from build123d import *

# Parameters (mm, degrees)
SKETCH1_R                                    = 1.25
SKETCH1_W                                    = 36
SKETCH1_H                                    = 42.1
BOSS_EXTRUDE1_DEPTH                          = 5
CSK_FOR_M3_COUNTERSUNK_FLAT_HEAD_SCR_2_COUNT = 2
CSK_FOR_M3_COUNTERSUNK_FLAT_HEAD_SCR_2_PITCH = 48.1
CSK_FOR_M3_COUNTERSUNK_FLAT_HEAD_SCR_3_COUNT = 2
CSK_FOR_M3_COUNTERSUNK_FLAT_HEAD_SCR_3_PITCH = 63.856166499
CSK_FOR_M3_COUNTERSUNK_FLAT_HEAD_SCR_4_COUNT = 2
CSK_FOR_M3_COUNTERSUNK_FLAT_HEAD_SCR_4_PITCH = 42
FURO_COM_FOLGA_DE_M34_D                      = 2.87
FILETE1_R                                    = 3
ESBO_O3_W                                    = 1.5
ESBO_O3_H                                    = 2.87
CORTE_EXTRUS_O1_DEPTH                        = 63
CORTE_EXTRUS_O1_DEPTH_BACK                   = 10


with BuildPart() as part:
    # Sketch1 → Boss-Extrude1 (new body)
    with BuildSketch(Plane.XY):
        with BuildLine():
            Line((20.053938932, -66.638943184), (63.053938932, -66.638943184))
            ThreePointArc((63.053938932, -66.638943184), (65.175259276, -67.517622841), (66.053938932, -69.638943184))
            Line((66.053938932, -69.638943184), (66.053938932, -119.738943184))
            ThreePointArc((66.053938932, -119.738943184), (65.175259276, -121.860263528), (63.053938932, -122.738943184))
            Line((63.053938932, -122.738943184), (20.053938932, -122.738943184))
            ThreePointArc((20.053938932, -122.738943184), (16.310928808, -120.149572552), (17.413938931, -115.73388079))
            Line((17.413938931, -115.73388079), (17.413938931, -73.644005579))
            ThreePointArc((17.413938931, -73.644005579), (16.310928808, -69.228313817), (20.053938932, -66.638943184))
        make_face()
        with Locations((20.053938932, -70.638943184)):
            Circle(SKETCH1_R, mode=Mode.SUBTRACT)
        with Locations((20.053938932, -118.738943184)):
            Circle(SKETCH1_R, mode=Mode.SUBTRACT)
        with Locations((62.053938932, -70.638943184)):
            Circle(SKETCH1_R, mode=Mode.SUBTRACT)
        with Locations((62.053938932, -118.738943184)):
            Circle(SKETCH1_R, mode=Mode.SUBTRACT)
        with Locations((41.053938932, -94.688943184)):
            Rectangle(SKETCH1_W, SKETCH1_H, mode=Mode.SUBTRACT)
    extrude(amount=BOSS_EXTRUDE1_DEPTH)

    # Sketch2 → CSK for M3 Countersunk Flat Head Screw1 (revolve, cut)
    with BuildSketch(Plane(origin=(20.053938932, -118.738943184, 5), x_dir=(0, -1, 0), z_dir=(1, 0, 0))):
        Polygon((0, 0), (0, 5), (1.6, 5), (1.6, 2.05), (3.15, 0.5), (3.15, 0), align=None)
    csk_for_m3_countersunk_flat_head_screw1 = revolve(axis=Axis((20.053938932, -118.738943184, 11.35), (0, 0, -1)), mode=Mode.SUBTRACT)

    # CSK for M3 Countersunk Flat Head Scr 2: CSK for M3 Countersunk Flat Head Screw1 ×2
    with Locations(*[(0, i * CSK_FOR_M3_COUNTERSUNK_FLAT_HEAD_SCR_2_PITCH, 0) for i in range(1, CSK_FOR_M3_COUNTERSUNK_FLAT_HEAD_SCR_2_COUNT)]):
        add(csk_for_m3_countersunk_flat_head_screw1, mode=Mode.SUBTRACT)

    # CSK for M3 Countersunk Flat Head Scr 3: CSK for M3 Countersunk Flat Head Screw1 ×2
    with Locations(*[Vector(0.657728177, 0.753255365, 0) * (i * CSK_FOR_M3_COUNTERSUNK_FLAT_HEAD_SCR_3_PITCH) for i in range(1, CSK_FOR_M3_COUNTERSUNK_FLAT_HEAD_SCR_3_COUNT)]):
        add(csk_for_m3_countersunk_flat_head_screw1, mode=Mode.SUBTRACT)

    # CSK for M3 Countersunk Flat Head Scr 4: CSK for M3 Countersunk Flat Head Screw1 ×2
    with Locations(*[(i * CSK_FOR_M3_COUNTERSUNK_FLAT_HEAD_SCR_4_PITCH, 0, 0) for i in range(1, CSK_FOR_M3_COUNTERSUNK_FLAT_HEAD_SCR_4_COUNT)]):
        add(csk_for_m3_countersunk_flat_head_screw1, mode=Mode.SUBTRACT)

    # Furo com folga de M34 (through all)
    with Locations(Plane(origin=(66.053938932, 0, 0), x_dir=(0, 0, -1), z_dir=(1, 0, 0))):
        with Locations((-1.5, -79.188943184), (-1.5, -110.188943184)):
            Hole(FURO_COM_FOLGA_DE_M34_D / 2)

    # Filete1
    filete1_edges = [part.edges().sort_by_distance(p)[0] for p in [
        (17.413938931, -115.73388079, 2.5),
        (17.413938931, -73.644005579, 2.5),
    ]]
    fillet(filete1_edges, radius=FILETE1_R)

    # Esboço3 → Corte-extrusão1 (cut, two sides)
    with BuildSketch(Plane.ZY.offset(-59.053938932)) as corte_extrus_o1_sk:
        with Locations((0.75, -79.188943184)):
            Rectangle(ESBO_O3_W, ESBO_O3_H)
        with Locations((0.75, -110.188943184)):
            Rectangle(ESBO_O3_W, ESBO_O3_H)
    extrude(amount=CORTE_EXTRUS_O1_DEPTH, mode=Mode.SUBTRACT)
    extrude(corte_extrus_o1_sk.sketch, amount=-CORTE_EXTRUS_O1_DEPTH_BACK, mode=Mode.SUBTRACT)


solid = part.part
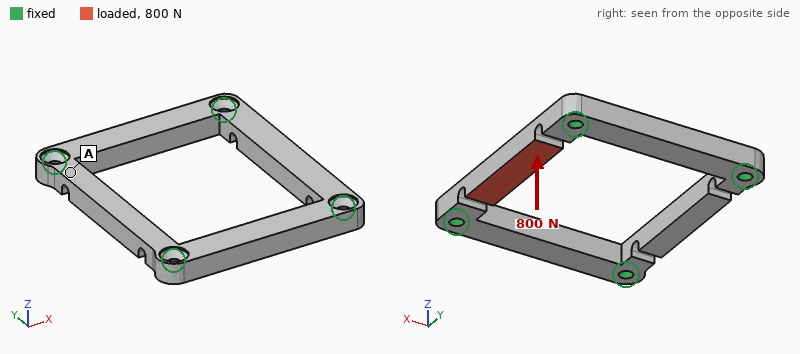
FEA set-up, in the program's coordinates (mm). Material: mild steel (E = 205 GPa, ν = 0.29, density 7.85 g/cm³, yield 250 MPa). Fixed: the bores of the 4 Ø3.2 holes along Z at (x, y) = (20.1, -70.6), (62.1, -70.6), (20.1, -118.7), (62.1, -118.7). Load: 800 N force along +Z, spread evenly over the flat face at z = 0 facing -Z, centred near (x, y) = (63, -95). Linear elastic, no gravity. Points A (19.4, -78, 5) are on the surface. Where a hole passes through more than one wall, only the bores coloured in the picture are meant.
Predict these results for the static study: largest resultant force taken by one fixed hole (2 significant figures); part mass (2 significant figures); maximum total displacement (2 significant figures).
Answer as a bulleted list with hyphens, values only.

- 410 N
- 44 g
- 35 µm
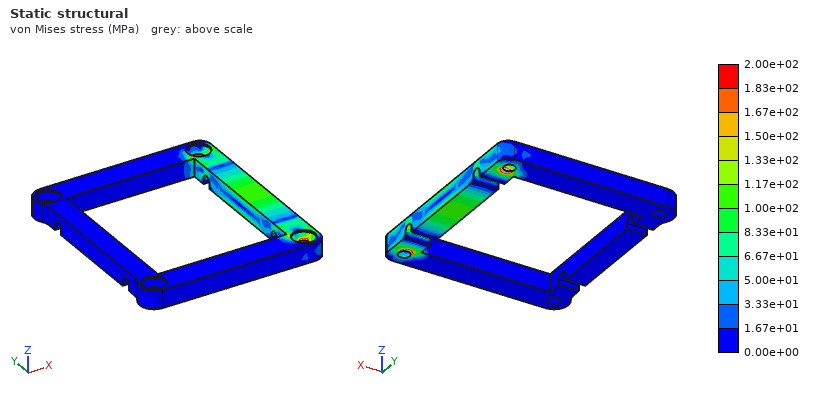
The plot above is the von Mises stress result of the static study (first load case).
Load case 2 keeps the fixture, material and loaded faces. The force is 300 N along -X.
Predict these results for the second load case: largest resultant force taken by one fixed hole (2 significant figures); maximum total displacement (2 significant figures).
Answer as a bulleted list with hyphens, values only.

- 150 N
- 12 µm
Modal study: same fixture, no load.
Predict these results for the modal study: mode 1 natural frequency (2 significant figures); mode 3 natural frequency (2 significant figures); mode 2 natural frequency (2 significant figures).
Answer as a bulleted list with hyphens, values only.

- 9400 Hz
- 11 kHz
- 9500 Hz
